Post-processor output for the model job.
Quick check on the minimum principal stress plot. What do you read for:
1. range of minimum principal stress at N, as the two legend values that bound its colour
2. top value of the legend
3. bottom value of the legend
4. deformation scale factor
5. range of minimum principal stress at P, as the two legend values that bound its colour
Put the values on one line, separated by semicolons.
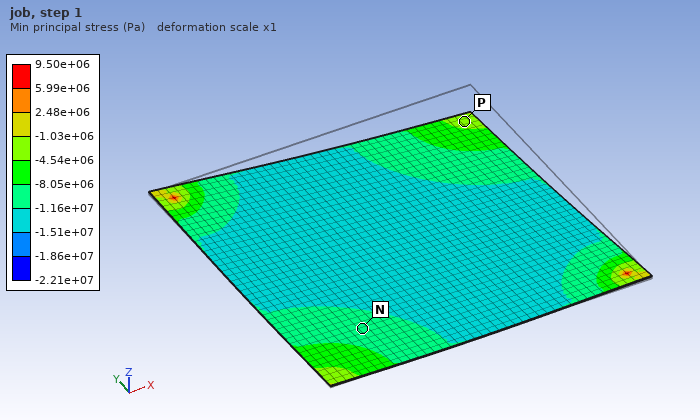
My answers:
-1.16e+07 to -8.05e+06 Pa; 9.50e+06 Pa; -2.21e+07 Pa; 1; -4.54e+06 to -1.03e+06 Pa
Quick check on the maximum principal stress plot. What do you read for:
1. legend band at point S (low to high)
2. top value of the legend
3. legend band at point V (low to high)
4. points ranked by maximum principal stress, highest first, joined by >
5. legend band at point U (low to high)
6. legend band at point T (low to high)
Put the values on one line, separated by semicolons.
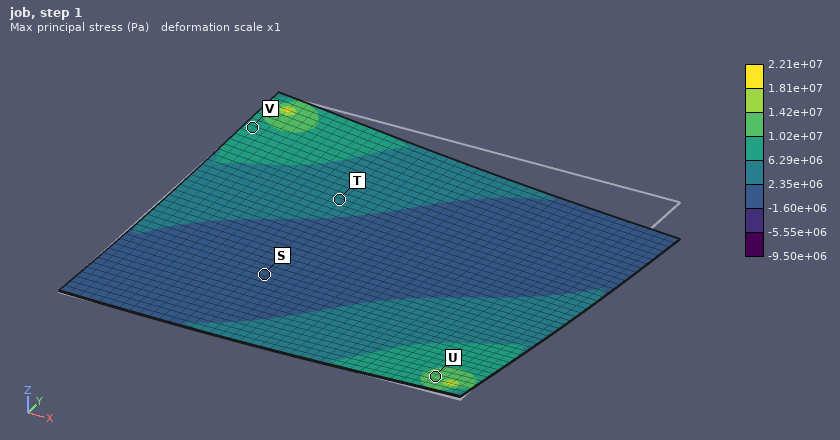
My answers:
-1.60e+06 to 2.35e+06 Pa; 2.21e+07 Pa; 6.29e+06 to 1.02e+07 Pa; U > V > T > S; 1.02e+07 to 1.42e+07 Pa; 2.35e+06 to 6.29e+06 Pa
